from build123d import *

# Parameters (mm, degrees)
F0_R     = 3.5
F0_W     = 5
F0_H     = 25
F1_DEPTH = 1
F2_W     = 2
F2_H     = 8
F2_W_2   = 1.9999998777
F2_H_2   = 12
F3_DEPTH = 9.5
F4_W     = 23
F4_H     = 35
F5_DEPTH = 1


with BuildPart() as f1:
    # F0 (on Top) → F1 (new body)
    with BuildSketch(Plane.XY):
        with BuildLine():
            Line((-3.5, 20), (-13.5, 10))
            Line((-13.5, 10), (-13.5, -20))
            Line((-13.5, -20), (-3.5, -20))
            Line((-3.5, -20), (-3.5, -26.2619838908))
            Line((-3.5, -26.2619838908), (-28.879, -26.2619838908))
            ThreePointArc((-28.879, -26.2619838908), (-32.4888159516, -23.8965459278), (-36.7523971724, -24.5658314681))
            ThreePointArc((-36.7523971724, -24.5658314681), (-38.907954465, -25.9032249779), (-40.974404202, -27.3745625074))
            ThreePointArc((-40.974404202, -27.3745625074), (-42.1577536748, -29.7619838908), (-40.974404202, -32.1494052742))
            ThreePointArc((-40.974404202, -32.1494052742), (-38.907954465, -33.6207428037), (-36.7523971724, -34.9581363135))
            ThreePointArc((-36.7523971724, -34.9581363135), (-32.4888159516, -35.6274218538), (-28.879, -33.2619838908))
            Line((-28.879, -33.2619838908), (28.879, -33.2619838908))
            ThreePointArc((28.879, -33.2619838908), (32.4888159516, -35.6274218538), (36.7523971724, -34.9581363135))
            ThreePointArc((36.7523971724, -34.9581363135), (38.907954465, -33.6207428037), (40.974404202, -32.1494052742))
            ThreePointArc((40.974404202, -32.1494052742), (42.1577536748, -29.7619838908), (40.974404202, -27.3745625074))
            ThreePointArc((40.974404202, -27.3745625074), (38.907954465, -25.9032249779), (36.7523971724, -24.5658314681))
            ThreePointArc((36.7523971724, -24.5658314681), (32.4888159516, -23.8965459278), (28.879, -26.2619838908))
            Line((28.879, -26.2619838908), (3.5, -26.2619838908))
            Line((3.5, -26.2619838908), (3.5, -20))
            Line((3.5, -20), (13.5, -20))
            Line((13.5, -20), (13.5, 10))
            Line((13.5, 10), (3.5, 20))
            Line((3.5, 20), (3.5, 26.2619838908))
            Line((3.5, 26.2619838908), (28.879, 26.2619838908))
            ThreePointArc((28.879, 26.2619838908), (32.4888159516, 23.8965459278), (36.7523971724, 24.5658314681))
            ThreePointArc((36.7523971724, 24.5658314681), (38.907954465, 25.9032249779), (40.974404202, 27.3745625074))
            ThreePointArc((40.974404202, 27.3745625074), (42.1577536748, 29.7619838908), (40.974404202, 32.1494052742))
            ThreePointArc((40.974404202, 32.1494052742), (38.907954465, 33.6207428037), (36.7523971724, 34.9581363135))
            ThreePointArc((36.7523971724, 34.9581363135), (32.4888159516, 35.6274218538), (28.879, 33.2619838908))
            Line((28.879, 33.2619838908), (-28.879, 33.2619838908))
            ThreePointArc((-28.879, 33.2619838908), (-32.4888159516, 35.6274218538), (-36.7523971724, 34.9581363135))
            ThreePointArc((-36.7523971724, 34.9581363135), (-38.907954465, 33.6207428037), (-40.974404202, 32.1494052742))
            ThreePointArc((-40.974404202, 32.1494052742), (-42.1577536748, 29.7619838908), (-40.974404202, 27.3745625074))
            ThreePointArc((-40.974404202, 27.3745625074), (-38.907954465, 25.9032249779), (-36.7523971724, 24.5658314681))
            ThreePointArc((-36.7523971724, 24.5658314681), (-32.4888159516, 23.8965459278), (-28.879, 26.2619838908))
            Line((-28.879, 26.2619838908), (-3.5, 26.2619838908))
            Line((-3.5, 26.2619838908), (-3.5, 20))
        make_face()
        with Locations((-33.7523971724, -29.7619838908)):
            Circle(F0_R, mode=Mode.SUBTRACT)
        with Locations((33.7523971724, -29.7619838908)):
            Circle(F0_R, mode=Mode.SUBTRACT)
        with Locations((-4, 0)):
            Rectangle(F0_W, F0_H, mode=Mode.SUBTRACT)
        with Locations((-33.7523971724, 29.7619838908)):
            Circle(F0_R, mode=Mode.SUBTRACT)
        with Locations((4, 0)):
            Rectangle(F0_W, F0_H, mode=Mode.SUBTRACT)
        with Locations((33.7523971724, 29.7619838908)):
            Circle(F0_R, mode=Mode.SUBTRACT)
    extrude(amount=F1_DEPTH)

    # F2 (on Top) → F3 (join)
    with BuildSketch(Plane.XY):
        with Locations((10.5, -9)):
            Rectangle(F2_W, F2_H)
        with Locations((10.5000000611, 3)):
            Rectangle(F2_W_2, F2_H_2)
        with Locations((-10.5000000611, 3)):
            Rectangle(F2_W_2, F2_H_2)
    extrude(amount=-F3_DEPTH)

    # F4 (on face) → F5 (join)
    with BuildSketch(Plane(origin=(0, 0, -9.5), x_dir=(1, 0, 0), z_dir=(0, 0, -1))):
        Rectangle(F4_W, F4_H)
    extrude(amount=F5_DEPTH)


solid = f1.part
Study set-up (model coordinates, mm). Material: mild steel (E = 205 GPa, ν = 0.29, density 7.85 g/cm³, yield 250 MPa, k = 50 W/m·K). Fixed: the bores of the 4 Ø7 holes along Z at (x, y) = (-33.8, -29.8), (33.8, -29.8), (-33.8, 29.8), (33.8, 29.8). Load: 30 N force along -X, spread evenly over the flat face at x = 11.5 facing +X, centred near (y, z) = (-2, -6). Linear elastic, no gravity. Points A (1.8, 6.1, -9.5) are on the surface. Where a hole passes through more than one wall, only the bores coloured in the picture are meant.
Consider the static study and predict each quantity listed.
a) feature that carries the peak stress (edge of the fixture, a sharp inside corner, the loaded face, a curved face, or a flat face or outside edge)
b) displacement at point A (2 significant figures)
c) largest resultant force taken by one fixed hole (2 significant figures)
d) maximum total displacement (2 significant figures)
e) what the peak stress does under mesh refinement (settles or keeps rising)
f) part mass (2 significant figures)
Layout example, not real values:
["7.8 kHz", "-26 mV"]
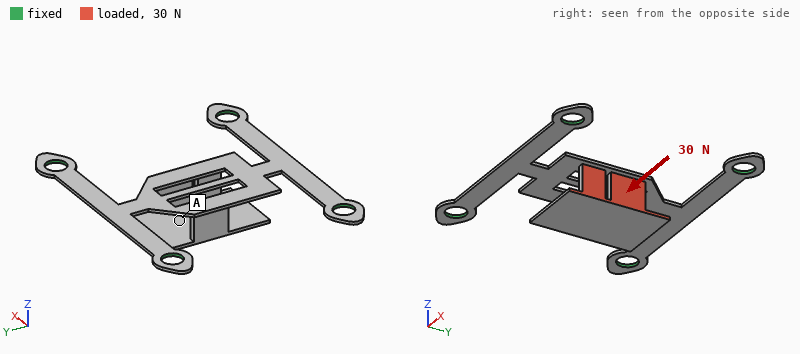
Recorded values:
["a sharp inside corner", "0.096 mm", "8.6 N", "0.15 mm", "keeps rising", "26 g"]
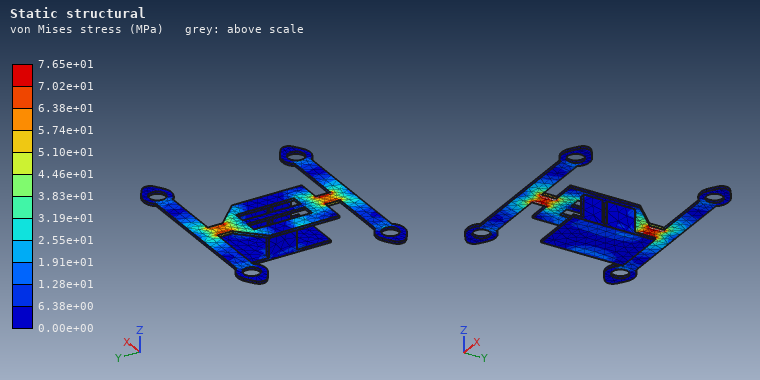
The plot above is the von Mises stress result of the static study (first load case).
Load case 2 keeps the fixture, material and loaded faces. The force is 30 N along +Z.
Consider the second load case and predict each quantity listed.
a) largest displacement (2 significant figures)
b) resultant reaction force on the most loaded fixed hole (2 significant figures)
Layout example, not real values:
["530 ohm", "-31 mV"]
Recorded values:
["0.48 mm", "12 N"]
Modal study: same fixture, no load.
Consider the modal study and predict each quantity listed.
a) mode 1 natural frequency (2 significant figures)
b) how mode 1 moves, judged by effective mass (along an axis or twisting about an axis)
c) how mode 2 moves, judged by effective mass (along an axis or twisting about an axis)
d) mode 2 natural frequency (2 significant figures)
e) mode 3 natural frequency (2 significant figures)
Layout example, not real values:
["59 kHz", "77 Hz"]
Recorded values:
["400 Hz", "along Z", "along X", "510 Hz", "800 Hz"]
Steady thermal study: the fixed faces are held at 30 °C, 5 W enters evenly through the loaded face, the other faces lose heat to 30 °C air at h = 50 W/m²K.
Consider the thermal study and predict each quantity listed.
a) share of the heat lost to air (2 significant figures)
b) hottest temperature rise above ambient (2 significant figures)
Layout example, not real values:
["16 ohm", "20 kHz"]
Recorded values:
["95 %", "41 K"]
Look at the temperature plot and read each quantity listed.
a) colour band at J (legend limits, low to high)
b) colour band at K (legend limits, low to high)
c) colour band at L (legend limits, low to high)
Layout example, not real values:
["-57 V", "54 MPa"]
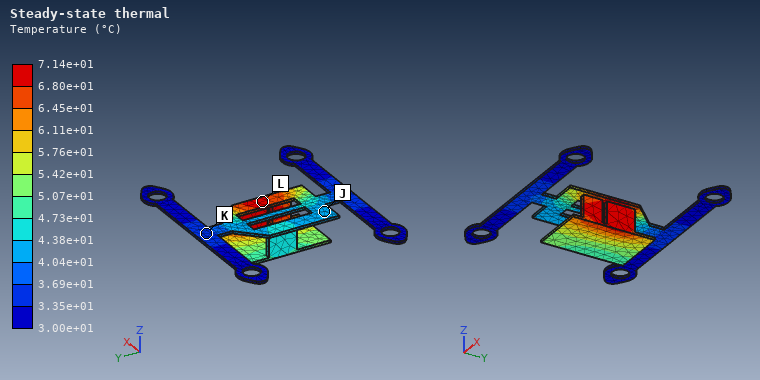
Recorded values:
["4.04e+01 to 4.38e+01 °C", "3.35e+01 to 3.69e+01 °C", "6.80e+01 to 7.14e+01 °C"]
